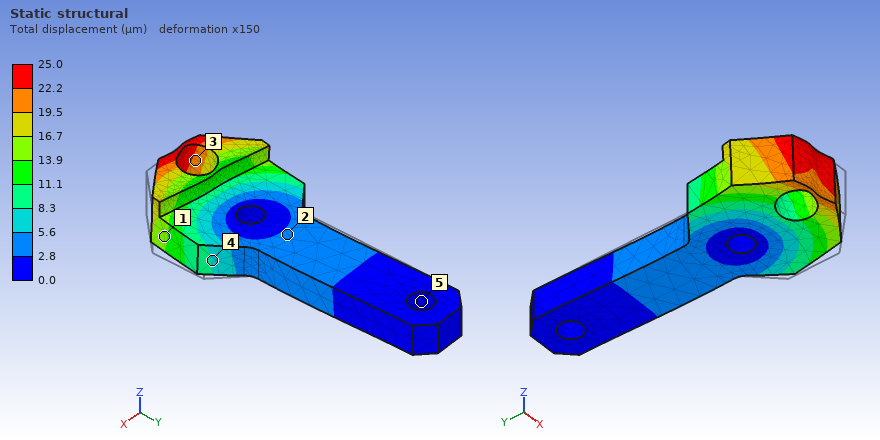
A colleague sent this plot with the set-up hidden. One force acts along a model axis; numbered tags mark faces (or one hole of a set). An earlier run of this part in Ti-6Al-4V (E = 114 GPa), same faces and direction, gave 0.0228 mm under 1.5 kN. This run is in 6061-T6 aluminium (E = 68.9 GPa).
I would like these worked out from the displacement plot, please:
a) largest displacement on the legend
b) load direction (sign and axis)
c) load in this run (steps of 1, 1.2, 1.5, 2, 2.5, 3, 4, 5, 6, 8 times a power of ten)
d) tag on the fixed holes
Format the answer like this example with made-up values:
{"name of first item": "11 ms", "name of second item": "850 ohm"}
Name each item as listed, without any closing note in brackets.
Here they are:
{"largest displacement on the legend": "25.0 µm", "load direction": "-X", "load in this run": "1 kN", "tag on the fixed holes": "5"}
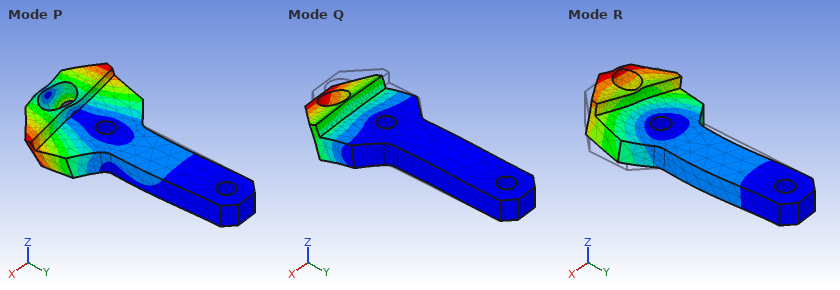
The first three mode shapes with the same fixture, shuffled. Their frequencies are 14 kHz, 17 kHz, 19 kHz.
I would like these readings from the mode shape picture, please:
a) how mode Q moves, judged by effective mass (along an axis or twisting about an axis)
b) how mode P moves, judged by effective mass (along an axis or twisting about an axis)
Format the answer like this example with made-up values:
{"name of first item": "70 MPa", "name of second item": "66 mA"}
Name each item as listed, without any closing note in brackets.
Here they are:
{"how mode Q moves, judged by effective mass": "along Z", "how mode P moves, judged by effective mass": "twisting about Y"}
